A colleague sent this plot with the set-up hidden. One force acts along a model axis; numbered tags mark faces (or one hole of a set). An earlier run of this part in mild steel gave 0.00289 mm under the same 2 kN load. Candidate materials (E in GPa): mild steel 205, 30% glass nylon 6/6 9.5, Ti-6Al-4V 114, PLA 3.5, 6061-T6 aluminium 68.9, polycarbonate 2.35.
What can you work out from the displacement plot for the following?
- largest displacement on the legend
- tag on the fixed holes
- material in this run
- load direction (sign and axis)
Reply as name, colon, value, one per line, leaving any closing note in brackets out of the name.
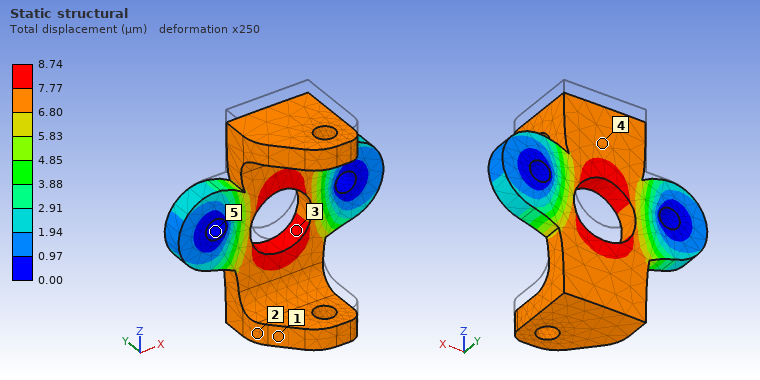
largest displacement on the legend: 8.74 µm
tag on the fixed holes: 5
material in this run: 6061-T6 aluminium
load direction: -Z
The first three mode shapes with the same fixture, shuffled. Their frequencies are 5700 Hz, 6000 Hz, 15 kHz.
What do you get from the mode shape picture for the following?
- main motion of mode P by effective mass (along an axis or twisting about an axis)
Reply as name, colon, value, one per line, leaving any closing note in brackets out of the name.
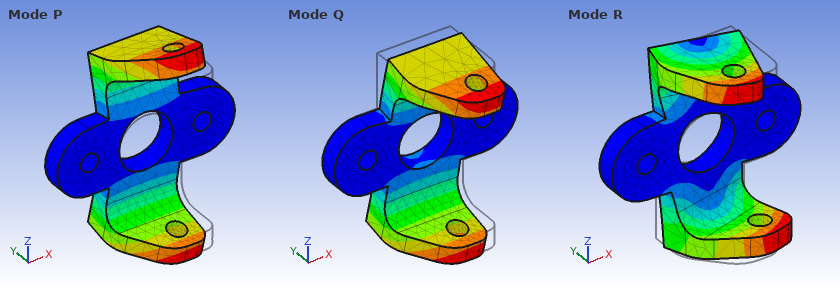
main motion of mode P by effective mass: along Y
